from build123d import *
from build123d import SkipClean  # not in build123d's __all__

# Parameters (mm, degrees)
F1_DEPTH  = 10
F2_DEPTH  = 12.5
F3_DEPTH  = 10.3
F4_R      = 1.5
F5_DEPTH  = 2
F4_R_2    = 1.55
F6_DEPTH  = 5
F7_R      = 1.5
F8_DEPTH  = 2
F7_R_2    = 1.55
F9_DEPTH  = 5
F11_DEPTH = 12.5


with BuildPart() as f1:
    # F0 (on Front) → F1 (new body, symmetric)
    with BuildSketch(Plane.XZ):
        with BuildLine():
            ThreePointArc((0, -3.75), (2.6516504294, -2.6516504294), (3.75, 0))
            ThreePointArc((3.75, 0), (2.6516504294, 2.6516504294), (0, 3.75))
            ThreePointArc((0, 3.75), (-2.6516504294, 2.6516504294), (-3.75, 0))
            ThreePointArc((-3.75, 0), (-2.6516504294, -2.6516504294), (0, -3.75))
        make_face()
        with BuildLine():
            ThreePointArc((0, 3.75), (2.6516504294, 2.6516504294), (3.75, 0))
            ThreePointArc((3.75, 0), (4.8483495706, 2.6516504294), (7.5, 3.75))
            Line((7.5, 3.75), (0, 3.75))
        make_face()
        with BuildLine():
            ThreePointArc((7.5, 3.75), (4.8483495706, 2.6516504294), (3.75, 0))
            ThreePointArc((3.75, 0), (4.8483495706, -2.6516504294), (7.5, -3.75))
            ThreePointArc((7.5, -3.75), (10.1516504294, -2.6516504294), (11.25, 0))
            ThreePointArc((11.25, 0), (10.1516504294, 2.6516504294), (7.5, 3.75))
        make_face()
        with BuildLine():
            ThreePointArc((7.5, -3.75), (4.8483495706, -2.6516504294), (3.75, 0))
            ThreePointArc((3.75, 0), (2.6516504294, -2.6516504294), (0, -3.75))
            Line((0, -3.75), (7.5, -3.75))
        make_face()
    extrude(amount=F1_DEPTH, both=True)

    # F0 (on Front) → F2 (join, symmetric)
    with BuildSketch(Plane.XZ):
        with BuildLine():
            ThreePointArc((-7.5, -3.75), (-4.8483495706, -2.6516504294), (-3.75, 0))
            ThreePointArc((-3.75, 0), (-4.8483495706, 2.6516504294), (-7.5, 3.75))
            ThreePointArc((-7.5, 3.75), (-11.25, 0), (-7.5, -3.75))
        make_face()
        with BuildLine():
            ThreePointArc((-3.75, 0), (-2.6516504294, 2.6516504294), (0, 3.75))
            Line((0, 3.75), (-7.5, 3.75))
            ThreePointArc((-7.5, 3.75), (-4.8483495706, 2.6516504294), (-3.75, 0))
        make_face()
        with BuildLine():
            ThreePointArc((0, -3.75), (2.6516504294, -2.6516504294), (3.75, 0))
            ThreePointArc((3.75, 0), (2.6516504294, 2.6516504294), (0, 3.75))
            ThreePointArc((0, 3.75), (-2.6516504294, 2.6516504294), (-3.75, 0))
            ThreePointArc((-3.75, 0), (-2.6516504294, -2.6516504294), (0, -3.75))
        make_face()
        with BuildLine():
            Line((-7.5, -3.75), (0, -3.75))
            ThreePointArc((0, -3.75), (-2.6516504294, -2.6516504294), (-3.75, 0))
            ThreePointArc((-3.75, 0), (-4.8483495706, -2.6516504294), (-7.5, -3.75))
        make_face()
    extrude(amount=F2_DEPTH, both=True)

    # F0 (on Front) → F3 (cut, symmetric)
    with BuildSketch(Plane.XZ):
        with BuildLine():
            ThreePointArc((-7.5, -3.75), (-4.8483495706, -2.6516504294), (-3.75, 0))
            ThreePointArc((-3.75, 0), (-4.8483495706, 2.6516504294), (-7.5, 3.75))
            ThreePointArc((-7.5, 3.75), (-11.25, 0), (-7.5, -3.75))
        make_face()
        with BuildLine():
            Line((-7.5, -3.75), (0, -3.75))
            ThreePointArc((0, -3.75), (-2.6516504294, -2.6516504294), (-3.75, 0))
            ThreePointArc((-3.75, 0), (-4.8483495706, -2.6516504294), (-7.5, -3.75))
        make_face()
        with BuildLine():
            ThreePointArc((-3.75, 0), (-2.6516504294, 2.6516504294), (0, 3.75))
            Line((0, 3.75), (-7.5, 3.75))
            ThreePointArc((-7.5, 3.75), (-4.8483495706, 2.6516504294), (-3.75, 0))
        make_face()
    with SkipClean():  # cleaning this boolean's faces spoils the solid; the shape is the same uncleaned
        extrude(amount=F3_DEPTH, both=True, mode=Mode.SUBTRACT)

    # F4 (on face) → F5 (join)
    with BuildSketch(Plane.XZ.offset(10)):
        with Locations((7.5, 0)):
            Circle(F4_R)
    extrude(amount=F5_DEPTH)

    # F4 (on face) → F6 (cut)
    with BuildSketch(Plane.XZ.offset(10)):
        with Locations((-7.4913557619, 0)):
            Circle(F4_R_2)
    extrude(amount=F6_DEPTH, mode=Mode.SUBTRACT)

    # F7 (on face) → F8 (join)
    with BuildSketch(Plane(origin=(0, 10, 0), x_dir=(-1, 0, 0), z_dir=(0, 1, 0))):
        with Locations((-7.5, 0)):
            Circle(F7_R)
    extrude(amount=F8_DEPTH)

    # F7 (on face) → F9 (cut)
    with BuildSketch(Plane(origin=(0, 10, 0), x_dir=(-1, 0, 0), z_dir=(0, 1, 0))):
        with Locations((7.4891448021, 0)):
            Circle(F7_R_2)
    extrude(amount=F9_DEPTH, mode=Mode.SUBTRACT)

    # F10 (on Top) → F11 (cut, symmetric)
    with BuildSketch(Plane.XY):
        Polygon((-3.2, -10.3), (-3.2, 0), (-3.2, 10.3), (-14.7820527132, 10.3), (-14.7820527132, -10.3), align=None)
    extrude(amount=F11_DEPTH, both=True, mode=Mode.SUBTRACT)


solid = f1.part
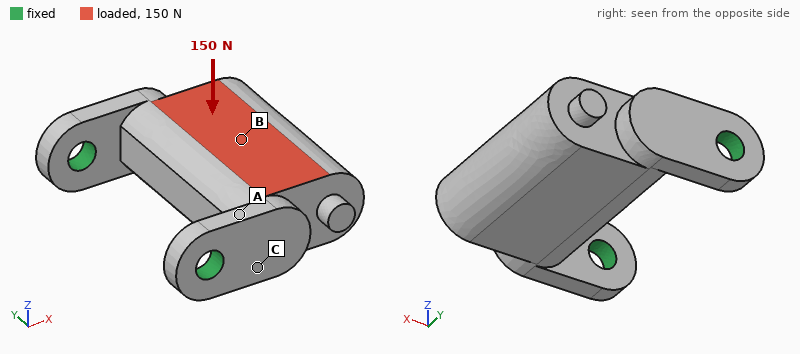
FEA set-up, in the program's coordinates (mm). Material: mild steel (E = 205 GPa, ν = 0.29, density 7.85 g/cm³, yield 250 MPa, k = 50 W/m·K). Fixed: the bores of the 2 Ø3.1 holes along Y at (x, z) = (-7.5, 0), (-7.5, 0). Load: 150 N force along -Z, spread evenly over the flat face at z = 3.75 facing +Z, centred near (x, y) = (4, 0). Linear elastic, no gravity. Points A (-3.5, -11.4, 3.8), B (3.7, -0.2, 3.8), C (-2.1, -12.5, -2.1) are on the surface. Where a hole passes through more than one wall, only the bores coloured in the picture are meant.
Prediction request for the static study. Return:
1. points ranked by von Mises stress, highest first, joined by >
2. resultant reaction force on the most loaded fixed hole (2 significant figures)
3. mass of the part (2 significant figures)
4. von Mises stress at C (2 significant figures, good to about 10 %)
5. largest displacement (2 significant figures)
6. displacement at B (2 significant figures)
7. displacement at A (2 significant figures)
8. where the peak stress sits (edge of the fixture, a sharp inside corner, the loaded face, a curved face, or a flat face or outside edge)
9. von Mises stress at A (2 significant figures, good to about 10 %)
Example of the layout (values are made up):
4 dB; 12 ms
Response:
A > C > B; 75 N; 19 g; 11 MPa; 6.9 µm; 4.2 µm; 1.4 µm; edge of the fixture; 25 MPa
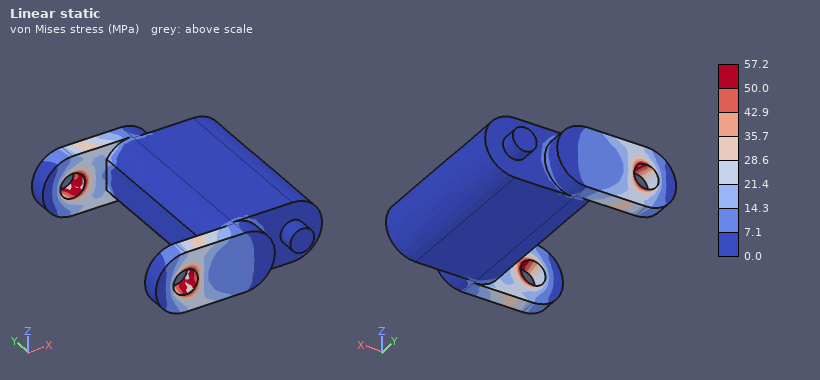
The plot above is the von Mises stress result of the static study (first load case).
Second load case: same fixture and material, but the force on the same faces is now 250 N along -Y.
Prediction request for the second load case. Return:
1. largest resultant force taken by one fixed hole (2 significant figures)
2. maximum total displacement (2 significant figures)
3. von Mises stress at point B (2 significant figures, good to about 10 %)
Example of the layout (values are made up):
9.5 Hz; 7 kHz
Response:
160 N; 2.0 µm; 6.0 MPa
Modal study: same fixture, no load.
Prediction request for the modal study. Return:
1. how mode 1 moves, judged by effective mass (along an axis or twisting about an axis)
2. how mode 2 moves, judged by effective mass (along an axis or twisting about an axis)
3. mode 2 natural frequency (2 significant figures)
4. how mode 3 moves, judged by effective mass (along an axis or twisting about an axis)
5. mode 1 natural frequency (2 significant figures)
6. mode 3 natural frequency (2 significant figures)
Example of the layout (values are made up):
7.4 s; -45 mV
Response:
along Z; along Y; 15 kHz; twisting about X; 7000 Hz; 24 kHz
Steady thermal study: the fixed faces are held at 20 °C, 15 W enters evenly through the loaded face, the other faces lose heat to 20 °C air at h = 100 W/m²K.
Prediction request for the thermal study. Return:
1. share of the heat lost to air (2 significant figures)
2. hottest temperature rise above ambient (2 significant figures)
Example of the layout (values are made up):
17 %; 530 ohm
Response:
29 %; 54 K
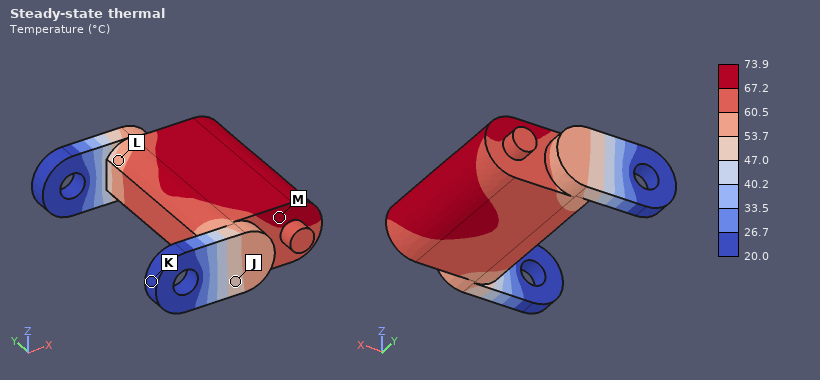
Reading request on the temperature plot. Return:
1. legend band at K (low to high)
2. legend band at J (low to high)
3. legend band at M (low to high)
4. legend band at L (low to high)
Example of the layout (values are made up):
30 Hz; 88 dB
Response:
20.0 to 26.7 °C; 47.0 to 53.7 °C; 67.2 to 73.9 °C; 53.7 to 60.5 °C
